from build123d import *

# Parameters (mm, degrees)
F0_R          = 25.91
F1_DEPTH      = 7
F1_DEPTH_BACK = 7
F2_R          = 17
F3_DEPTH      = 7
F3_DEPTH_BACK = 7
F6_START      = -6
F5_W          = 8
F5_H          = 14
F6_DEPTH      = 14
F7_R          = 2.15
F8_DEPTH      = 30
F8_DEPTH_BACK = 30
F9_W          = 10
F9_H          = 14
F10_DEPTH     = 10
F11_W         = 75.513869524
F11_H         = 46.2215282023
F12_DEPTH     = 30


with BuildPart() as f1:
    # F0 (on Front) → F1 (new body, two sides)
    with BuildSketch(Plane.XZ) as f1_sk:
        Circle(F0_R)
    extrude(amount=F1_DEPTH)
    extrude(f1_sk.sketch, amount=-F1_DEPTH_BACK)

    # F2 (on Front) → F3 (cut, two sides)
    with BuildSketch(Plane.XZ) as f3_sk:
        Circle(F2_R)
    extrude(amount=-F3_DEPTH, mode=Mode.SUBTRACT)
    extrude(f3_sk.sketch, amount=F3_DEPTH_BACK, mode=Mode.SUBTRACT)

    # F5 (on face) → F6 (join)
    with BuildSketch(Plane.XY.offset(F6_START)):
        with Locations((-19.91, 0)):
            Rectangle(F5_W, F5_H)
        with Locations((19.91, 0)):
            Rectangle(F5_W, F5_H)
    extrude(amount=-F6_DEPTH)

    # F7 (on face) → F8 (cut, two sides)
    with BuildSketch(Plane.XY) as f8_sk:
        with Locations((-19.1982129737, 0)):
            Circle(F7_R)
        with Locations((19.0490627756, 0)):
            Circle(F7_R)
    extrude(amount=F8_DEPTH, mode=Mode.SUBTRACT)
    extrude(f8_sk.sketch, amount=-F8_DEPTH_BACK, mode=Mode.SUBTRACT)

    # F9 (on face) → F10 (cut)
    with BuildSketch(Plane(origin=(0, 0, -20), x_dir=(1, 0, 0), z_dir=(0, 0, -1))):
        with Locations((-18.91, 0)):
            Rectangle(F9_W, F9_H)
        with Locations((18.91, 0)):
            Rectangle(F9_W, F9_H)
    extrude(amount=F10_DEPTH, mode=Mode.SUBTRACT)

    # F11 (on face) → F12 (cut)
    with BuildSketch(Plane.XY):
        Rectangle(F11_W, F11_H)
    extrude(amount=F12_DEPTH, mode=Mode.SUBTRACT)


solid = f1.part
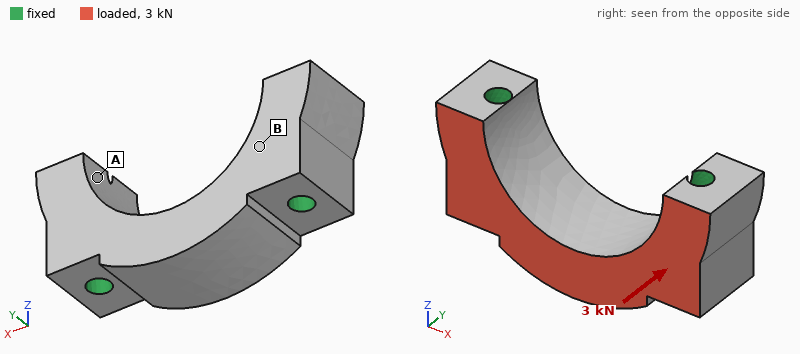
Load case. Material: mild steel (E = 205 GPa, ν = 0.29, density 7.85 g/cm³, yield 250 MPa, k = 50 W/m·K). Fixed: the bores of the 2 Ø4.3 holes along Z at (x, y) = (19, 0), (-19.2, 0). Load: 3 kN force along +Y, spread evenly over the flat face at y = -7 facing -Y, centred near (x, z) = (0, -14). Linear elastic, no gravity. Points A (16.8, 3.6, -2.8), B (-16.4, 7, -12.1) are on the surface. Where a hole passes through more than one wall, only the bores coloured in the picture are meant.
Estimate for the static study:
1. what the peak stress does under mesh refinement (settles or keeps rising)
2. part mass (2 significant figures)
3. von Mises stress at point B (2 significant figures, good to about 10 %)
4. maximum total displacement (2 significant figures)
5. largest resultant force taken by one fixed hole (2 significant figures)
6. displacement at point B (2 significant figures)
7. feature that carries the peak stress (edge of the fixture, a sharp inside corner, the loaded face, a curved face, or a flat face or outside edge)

keeps rising
68 g
11 MPa
3.1 µm
1.5 kN
0.49 µm
edge of the fixture
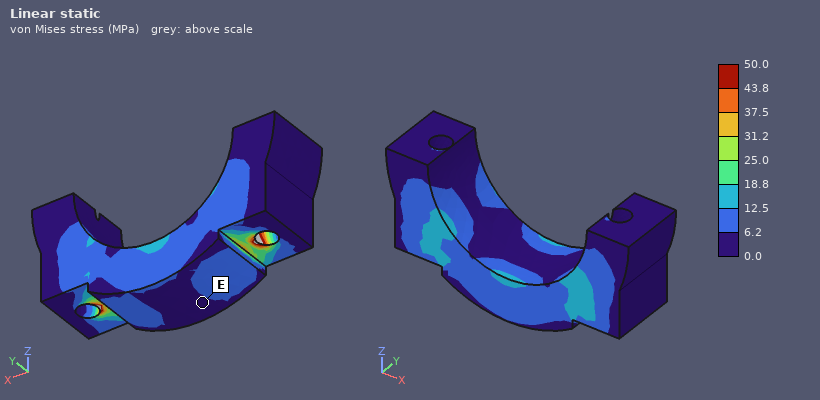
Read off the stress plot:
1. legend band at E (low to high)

0.0 to 6.2 MPa
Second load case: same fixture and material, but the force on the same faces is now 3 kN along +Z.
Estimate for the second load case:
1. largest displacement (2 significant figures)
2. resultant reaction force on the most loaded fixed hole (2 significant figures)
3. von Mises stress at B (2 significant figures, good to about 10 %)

4.2 µm
1.6 kN
6.5 MPa
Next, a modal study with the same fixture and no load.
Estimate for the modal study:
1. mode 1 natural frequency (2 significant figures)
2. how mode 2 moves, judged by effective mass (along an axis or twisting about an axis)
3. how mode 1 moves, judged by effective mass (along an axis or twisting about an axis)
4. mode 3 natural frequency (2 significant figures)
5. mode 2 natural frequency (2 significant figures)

23 kHz
along Z
along Y
45 kHz
34 kHz
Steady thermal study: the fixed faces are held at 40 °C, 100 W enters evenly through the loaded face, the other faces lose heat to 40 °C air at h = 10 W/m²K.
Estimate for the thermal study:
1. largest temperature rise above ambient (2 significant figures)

59 K
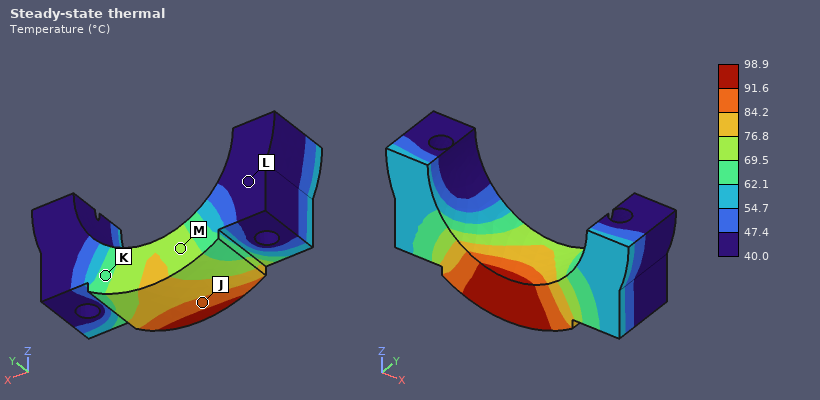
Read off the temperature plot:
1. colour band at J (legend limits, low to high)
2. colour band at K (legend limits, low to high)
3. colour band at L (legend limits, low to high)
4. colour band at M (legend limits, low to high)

84.2 to 91.6 °C
62.1 to 69.5 °C
40.0 to 47.4 °C
69.5 to 76.8 °C
